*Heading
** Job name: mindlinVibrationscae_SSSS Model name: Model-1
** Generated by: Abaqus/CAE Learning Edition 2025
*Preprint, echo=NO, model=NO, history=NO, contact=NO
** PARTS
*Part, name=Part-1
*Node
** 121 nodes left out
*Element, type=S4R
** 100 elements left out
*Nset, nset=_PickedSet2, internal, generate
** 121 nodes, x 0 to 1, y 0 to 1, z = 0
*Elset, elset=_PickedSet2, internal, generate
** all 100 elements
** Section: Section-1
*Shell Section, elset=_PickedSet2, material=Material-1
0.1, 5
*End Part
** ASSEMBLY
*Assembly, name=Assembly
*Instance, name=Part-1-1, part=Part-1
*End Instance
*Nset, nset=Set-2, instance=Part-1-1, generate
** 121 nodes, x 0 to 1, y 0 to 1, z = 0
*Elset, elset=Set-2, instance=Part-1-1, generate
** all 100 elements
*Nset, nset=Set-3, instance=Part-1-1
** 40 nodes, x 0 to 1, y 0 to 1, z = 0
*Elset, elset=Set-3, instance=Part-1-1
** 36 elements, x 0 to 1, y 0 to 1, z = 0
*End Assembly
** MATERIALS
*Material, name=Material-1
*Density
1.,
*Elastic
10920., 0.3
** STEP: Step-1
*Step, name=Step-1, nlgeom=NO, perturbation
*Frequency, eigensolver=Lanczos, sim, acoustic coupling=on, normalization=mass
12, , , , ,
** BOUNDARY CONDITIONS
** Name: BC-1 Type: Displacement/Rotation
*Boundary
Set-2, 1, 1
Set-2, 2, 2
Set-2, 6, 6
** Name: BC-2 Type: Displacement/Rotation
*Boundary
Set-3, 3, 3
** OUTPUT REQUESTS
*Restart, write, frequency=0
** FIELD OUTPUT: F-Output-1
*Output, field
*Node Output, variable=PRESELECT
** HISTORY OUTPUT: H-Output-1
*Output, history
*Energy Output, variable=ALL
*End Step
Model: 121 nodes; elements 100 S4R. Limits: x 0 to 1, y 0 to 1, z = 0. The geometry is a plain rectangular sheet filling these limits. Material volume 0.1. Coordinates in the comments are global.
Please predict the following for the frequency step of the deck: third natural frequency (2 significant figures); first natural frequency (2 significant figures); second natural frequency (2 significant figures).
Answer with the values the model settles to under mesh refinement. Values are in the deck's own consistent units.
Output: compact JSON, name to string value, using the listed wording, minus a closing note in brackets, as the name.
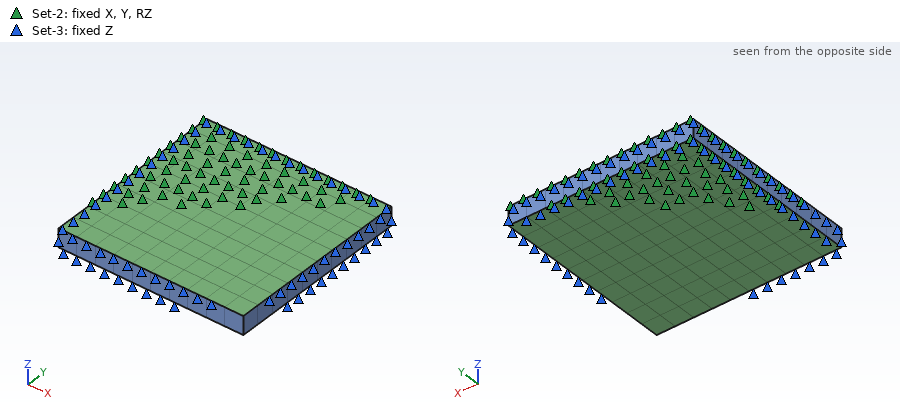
{"third natural frequency": "23 cycles per unit time", "first natural frequency": "9.3 cycles per unit time", "second natural frequency": "23 cycles per unit time"}
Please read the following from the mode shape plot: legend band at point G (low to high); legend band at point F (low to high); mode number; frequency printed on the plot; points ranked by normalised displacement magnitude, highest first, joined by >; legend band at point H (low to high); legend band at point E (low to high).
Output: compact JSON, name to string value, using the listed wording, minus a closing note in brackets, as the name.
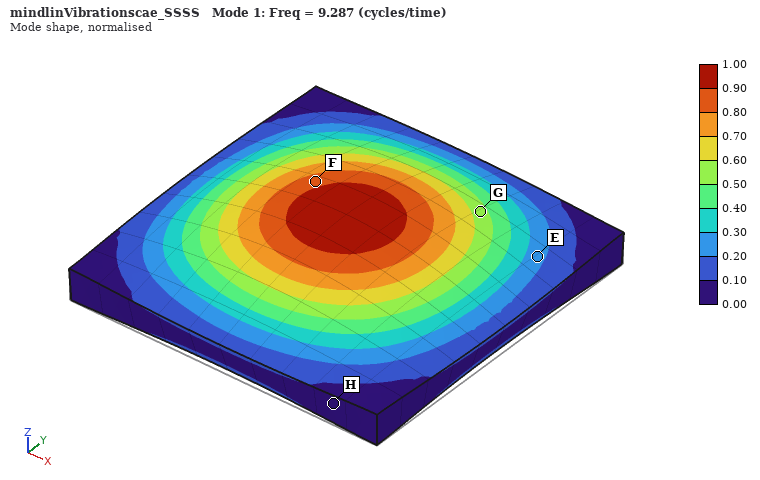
{"legend band at point G": "0.50 to 0.60", "legend band at point F": "0.80 to 0.90", "mode number": "1", "frequency printed on the plot": "9.287", "points ranked by normalised displacement magnitude, highest first, joined by >": "F > G > E > H", "legend band at point H": "0.00 to 0.10", "legend band at point E": "0.20 to 0.30"}
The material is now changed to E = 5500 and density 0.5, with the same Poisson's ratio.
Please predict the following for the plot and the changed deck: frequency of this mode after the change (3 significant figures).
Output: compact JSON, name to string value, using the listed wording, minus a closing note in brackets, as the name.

{"frequency of this mode after the change": "9.32"}
